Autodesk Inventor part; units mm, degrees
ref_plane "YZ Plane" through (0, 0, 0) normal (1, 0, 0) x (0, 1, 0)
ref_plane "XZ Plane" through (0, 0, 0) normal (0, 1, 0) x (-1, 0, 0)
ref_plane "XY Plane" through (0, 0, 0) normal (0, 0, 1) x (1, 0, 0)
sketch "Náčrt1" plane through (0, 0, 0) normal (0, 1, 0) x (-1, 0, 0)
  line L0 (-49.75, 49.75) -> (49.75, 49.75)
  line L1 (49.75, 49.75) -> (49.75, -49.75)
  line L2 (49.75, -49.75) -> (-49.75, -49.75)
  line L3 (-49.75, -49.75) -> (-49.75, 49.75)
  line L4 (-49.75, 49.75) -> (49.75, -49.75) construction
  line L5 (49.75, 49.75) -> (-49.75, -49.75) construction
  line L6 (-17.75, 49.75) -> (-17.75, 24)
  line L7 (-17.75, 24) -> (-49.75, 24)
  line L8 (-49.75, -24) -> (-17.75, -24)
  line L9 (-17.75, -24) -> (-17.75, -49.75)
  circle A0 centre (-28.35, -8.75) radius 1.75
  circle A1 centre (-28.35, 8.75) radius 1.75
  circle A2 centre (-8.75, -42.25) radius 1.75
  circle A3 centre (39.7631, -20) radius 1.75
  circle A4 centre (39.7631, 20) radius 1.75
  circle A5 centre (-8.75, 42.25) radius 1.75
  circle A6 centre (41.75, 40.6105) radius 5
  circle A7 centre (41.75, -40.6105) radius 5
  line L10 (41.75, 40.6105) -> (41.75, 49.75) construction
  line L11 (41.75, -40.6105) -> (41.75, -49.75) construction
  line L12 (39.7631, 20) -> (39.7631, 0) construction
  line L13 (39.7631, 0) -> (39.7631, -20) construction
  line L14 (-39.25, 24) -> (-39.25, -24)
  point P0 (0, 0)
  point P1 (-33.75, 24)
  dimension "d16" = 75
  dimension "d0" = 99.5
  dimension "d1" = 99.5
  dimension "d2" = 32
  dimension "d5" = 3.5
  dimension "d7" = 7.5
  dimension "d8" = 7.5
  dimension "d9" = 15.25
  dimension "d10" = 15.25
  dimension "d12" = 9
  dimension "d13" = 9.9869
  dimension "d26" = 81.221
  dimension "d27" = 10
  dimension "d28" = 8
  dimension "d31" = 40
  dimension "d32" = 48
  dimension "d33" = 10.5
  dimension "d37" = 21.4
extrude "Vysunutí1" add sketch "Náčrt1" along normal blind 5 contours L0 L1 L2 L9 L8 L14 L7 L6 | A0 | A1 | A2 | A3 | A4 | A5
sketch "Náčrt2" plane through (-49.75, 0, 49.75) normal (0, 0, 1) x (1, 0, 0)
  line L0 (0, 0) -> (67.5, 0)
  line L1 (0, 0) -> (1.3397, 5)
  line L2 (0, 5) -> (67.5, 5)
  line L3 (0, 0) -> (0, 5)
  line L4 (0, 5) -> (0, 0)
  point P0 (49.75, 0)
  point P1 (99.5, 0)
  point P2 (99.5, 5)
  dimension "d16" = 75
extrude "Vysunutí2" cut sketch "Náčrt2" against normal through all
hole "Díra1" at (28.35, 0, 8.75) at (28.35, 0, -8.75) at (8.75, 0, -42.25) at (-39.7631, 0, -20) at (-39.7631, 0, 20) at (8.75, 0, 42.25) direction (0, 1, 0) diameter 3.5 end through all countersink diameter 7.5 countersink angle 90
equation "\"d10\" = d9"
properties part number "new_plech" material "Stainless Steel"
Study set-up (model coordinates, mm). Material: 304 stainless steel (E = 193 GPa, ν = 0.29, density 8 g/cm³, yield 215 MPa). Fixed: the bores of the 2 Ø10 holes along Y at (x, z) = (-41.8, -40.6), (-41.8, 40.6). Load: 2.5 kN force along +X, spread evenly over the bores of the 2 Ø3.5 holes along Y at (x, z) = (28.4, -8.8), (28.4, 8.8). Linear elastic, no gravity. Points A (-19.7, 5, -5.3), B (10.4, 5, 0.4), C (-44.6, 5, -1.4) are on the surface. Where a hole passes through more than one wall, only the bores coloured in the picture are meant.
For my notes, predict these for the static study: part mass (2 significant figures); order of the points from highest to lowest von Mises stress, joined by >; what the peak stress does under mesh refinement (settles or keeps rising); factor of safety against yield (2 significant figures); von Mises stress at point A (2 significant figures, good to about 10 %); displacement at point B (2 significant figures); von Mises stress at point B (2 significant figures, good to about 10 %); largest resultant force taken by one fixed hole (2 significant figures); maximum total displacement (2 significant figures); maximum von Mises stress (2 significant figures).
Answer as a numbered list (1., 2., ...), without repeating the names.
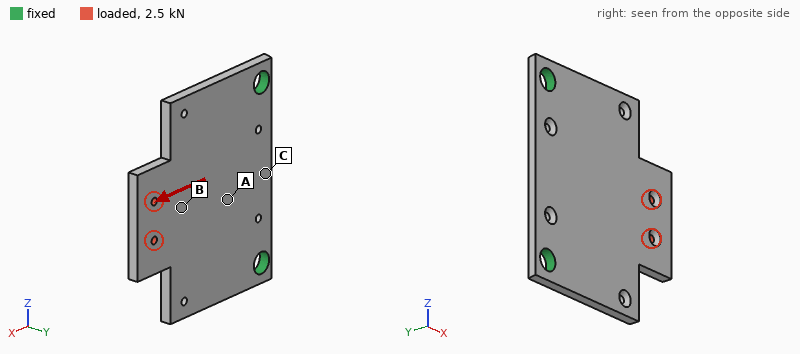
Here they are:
1. 300 g
2. B > A > C
3. settles
4. 3.0
5. 8.7 MPa
6. 22 µm
7. 18 MPa
8. 1.3 kN
9. 53 µm
10. 73 MPa
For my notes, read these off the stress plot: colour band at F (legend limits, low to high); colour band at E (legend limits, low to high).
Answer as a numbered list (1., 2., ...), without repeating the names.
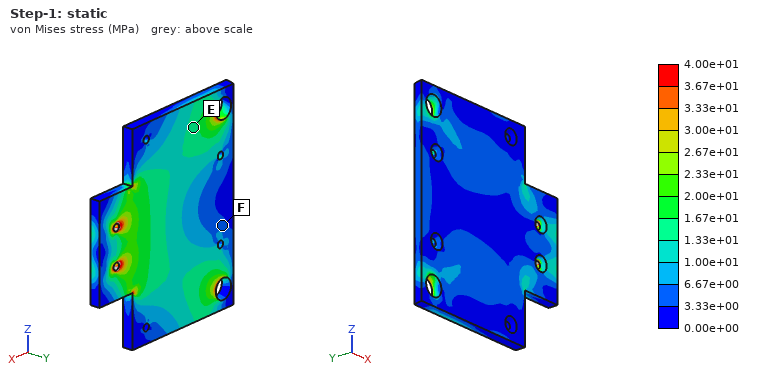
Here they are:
1. 3.33e+00 to 6.67e+00 MPa
2. 1.33e+01 to 1.67e+01 MPa
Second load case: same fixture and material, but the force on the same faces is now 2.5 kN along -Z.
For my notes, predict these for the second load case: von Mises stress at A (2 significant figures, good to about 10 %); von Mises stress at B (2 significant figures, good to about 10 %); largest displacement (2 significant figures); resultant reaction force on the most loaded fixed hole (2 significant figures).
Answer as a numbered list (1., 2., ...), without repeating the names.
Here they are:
1. 11 MPa
2. 20 MPa
3. 20 µm
4. 2.4 kN
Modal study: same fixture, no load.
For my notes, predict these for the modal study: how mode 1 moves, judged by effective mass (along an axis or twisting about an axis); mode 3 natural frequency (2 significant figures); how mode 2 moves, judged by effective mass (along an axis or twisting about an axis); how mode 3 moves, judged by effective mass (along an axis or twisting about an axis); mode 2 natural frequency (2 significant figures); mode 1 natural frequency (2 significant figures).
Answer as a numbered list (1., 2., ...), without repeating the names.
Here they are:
1. along Y
2. 3300 Hz
3. twisting about X
4. along Y
5. 1900 Hz
6. 680 Hz
